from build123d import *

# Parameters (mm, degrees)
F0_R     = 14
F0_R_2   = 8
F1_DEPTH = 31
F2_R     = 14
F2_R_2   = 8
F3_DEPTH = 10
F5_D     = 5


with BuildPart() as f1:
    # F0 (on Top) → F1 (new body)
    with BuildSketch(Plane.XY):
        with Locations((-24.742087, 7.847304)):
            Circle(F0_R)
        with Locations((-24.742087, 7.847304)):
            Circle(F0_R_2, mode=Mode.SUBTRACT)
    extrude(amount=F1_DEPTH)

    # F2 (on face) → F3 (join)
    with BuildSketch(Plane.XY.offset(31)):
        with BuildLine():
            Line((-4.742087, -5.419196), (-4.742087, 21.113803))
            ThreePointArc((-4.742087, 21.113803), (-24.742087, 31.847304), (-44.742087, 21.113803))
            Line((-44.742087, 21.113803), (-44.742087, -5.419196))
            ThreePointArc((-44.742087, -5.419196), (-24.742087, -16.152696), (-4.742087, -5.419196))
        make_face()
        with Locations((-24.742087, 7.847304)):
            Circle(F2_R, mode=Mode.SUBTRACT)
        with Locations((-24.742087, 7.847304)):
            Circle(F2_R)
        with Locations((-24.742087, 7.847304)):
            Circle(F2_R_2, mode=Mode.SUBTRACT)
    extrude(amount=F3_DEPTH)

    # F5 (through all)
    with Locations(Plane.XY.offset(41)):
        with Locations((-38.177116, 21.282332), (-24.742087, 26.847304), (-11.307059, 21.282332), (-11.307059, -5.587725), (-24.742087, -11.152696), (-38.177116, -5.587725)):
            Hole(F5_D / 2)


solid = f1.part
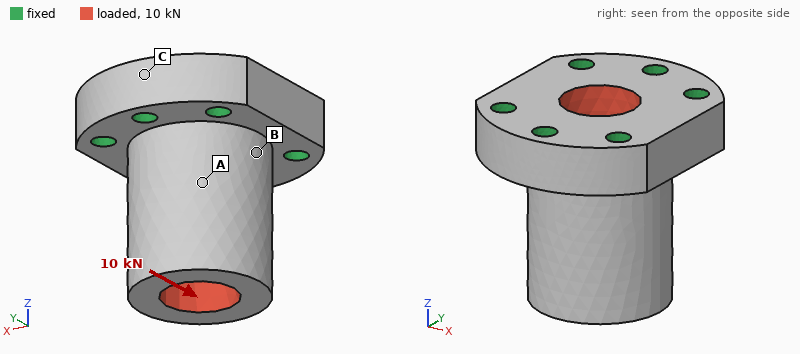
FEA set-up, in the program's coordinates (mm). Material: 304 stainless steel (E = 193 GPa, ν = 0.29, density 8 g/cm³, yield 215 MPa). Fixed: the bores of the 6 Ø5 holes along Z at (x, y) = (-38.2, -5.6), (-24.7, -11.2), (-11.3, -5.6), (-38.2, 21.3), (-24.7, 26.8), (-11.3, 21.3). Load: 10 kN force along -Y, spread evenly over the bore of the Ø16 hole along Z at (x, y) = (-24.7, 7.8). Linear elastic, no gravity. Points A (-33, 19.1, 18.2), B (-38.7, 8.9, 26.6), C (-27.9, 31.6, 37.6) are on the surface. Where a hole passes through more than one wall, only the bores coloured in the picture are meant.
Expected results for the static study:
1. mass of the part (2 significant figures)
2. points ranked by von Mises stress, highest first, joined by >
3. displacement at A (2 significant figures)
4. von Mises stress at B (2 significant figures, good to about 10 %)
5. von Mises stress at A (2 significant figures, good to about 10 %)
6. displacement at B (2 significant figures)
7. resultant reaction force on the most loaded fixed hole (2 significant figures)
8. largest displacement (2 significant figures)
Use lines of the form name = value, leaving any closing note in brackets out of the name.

mass of the part = 210 g
points ranked by von Mises stress, highest first, joined by > = B > A > C
displacement at A = 9.1 µm
von Mises stress at B = 30 MPa
von Mises stress at A = 21 MPa
displacement at B = 3.1 µm
resultant reaction force on the most loaded fixed hole = 3.0 kN
largest displacement = 18 µm
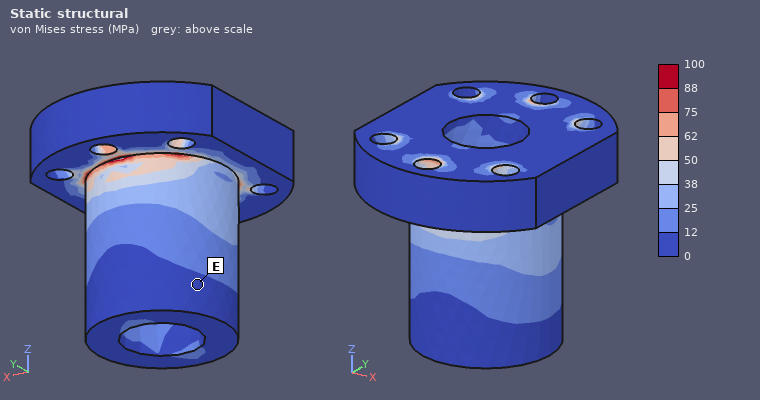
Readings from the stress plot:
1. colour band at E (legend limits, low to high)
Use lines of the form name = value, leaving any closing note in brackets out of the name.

colour band at E = 0 to 12 MPa
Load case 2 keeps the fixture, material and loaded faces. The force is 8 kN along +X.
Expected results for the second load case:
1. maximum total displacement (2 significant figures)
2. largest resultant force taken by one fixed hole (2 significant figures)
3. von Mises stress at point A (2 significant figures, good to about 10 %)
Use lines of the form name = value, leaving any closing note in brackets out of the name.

maximum total displacement = 17 µm
largest resultant force taken by one fixed hole = 2.9 kN
von Mises stress at point A = 19 MPa
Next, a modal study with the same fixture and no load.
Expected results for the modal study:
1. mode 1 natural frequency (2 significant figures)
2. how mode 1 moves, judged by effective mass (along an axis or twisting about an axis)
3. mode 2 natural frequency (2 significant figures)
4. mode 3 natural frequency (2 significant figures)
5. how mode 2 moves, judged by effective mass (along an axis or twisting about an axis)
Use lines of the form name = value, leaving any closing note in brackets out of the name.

mode 1 natural frequency = 11 kHz
how mode 1 moves, judged by effective mass = along X
mode 2 natural frequency = 12 kHz
mode 3 natural frequency = 22 kHz
how mode 2 moves, judged by effective mass = along Y
